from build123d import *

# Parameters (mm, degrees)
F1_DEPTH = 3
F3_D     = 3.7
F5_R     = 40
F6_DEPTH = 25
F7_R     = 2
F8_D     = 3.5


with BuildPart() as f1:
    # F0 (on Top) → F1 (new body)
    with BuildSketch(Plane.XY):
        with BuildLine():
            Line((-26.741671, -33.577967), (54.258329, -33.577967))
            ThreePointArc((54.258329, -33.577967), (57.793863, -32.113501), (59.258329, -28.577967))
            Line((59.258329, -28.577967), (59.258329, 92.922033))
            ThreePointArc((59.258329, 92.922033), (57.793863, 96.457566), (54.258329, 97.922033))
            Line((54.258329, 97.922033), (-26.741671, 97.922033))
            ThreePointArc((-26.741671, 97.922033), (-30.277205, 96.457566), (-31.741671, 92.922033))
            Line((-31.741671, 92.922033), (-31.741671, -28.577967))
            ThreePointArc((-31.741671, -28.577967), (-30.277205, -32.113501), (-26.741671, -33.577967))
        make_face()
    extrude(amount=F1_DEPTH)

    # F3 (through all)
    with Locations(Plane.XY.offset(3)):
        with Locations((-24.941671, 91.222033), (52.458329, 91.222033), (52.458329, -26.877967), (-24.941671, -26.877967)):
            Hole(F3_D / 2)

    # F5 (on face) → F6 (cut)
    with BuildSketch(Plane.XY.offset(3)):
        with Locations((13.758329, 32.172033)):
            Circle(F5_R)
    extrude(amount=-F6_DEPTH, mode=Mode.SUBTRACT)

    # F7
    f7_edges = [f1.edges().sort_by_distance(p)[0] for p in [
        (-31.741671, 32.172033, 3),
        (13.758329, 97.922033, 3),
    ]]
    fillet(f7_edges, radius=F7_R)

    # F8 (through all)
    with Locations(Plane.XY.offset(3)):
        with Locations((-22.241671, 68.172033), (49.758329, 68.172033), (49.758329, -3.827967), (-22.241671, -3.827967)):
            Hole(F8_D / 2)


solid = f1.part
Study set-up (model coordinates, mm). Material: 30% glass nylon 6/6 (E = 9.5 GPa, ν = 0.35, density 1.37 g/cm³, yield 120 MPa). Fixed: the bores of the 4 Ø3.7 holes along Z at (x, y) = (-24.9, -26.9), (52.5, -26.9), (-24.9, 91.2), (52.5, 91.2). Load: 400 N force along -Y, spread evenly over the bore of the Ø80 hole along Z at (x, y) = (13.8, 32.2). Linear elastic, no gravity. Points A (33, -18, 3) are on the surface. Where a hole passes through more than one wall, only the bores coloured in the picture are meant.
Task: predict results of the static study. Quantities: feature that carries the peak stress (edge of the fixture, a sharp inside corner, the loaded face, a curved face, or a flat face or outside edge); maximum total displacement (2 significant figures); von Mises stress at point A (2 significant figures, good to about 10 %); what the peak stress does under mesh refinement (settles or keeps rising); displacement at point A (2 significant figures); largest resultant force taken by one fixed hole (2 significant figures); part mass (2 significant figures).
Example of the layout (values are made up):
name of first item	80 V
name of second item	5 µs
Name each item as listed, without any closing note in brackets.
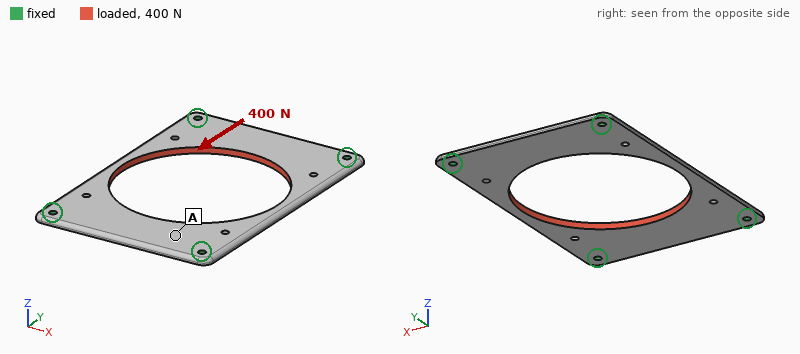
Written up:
feature that carries the peak stress	edge of the fixture
maximum total displacement	14 µm
von Mises stress at point A	1.1 MPa
what the peak stress does under mesh refinement	keeps rising
displacement at point A	9.6 µm
largest resultant force taken by one fixed hole	110 N
part mass	28 g
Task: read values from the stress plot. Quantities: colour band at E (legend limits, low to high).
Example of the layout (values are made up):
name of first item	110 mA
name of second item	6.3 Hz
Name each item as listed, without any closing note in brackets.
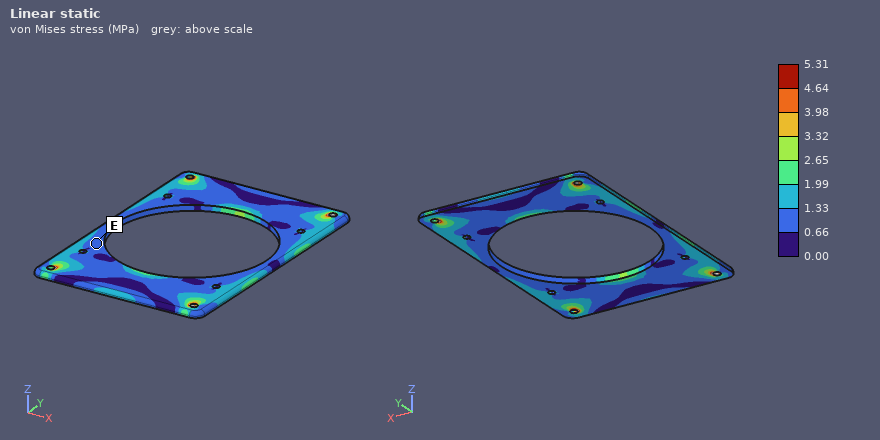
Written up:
colour band at E	0.66 to 1.33 MPa
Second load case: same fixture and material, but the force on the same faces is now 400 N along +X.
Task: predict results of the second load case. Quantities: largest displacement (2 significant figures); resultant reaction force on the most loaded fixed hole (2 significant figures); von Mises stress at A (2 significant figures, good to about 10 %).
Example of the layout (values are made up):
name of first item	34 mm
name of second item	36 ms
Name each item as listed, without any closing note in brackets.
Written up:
largest displacement	56 µm
resultant reaction force on the most loaded fixed hole	100 N
von Mises stress at A	1.7 MPa
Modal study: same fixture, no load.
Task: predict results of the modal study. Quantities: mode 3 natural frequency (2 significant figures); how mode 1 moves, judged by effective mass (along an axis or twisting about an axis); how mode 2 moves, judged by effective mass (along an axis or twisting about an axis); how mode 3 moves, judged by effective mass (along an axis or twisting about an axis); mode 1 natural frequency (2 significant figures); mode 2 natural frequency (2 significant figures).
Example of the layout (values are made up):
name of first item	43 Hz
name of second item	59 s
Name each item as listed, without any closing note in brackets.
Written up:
mode 3 natural frequency	1100 Hz
how mode 1 moves, judged by effective mass	along Z
how mode 2 moves, judged by effective mass	twisting about Y
how mode 3 moves, judged by effective mass	twisting about X
mode 1 natural frequency	720 Hz
mode 2 natural frequency	810 Hz
